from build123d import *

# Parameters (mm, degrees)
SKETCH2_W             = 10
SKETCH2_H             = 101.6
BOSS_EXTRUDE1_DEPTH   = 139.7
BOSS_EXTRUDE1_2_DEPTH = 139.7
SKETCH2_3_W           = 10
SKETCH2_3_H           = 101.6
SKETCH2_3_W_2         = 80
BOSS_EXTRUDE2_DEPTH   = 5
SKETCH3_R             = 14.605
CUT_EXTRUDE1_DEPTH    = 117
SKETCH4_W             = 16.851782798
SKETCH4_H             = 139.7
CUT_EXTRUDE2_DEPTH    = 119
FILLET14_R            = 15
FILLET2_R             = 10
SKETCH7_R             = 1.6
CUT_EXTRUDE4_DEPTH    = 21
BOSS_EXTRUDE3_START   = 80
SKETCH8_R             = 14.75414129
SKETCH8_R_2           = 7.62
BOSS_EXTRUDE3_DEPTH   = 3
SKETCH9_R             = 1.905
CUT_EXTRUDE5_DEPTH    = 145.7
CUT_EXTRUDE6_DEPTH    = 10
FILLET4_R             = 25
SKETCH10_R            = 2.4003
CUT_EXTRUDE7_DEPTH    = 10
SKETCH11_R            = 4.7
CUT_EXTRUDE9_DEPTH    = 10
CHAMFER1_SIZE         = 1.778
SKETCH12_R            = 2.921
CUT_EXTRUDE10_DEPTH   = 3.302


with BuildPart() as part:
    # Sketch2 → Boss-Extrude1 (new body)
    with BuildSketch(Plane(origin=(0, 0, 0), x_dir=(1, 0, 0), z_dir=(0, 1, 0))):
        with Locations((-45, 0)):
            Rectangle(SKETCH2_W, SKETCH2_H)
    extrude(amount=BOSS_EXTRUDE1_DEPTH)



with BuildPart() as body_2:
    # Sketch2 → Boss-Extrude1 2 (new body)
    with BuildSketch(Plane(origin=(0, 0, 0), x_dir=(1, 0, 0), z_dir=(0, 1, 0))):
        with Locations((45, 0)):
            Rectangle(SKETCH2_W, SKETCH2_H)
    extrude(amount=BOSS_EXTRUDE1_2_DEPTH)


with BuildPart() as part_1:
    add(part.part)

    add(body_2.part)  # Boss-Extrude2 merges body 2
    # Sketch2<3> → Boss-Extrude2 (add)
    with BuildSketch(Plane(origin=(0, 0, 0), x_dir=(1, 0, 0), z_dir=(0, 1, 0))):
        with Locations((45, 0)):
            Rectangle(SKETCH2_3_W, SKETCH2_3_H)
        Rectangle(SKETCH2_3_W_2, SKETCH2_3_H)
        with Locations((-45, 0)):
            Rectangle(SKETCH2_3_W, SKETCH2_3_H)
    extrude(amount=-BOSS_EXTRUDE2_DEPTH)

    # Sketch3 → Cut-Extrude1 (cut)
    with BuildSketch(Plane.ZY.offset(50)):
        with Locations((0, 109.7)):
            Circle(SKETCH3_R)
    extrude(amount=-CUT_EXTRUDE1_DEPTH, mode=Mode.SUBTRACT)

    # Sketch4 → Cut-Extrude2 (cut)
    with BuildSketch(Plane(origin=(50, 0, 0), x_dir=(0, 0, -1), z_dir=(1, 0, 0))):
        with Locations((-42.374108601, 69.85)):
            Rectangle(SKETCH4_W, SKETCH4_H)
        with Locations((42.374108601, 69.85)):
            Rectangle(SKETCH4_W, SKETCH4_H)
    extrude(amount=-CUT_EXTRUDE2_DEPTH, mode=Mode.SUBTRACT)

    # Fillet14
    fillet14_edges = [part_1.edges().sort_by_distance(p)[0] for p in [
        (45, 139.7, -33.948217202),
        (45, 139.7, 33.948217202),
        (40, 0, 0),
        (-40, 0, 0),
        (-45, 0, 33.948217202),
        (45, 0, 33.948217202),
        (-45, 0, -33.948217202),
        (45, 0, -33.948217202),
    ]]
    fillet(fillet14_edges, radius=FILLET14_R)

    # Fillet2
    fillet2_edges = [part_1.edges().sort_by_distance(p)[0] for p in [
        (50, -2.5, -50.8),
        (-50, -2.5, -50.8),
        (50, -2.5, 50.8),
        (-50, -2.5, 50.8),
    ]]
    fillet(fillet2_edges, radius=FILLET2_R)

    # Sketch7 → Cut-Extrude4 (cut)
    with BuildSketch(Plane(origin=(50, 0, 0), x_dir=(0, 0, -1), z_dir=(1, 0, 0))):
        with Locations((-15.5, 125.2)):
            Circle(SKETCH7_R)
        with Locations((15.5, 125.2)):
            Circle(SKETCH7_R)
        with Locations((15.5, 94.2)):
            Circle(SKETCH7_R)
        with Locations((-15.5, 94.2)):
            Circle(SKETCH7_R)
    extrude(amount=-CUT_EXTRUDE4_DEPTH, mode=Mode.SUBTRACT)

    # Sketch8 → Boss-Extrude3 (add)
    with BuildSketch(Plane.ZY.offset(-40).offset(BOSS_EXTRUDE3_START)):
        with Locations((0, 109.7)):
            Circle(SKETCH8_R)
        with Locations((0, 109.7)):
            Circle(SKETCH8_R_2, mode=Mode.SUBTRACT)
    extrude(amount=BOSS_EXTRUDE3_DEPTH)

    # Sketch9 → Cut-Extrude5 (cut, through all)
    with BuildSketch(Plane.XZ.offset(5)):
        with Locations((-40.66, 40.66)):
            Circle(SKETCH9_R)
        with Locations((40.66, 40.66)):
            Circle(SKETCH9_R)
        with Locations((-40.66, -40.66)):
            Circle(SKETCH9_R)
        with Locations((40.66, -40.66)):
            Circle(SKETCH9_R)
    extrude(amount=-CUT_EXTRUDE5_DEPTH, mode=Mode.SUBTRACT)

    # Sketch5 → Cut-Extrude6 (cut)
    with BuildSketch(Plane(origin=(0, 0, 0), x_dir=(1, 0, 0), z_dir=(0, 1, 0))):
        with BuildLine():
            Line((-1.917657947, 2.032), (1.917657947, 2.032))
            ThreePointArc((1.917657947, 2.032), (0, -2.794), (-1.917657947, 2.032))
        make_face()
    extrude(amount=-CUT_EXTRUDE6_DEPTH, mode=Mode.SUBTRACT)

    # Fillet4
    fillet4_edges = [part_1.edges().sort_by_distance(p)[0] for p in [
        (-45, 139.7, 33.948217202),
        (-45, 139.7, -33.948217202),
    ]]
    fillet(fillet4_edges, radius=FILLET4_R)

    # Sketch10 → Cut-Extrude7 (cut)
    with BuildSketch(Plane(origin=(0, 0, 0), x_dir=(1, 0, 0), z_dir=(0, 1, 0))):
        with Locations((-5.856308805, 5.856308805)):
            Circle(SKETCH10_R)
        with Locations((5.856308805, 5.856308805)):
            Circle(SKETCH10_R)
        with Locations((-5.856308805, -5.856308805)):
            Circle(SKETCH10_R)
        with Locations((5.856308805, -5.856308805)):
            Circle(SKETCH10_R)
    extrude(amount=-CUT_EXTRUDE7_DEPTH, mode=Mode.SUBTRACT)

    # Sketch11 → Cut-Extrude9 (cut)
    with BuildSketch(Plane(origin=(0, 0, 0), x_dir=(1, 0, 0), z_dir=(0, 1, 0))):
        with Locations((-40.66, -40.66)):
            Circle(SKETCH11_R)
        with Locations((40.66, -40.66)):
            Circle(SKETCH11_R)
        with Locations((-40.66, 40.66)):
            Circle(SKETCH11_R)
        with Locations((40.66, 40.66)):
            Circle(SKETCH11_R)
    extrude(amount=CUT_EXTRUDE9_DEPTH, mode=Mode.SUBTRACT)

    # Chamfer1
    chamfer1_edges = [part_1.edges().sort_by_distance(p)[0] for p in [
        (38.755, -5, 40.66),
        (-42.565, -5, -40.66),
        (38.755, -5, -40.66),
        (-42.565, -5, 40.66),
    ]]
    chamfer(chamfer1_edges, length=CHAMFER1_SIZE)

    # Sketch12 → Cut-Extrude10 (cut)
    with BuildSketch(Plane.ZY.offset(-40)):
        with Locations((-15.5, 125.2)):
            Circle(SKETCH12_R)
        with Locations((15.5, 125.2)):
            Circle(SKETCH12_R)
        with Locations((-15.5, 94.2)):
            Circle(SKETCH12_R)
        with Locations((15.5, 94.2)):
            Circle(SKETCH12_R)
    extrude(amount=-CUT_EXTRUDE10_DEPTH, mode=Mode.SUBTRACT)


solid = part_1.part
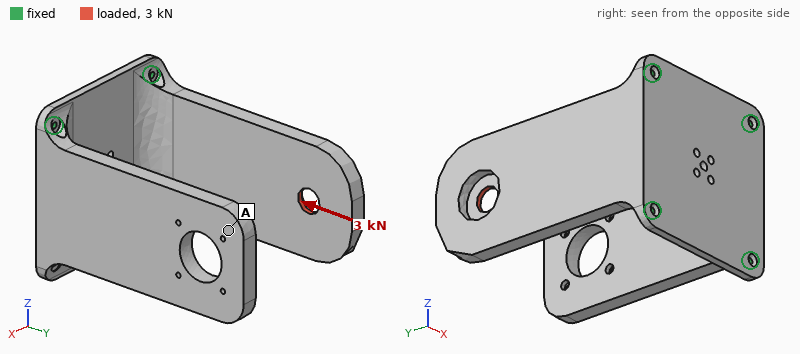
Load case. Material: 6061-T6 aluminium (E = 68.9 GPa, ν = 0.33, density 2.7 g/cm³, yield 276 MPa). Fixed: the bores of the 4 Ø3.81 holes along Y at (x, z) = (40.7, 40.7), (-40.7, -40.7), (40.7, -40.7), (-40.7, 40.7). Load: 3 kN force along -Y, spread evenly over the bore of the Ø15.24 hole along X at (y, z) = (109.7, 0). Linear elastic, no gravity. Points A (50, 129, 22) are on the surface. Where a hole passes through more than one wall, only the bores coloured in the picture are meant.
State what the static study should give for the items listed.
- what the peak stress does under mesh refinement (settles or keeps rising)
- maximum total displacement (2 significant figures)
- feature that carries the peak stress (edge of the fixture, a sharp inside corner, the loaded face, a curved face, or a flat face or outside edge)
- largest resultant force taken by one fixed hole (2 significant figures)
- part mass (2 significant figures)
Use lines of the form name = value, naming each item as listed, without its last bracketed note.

what the peak stress does under mesh refinement = keeps rising
maximum total displacement = 0.18 mm
feature that carries the peak stress = edge of the fixture
largest resultant force taken by one fixed hole = 1.7 kN
part mass = 630 g
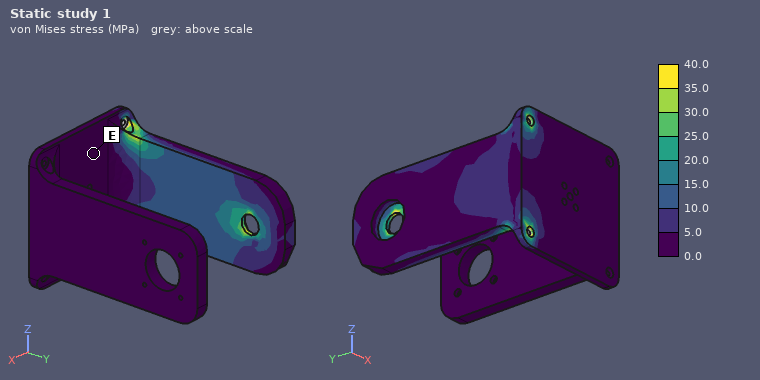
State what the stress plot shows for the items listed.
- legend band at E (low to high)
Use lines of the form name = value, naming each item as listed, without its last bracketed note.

legend band at E = 0.0 to 5.0 MPa
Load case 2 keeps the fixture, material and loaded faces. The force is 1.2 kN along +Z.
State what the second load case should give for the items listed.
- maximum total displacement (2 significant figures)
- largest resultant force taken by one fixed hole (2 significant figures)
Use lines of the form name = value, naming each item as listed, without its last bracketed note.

maximum total displacement = 0.11 mm
largest resultant force taken by one fixed hole = 1.8 kN
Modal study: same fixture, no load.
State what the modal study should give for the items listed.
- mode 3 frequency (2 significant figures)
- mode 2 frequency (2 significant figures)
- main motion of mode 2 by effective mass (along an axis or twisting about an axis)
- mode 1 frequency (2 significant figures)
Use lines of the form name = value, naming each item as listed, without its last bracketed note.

mode 3 frequency = 1700 Hz
mode 2 frequency = 360 Hz
main motion of mode 2 by effective mass = along X
mode 1 frequency = 300 Hz
